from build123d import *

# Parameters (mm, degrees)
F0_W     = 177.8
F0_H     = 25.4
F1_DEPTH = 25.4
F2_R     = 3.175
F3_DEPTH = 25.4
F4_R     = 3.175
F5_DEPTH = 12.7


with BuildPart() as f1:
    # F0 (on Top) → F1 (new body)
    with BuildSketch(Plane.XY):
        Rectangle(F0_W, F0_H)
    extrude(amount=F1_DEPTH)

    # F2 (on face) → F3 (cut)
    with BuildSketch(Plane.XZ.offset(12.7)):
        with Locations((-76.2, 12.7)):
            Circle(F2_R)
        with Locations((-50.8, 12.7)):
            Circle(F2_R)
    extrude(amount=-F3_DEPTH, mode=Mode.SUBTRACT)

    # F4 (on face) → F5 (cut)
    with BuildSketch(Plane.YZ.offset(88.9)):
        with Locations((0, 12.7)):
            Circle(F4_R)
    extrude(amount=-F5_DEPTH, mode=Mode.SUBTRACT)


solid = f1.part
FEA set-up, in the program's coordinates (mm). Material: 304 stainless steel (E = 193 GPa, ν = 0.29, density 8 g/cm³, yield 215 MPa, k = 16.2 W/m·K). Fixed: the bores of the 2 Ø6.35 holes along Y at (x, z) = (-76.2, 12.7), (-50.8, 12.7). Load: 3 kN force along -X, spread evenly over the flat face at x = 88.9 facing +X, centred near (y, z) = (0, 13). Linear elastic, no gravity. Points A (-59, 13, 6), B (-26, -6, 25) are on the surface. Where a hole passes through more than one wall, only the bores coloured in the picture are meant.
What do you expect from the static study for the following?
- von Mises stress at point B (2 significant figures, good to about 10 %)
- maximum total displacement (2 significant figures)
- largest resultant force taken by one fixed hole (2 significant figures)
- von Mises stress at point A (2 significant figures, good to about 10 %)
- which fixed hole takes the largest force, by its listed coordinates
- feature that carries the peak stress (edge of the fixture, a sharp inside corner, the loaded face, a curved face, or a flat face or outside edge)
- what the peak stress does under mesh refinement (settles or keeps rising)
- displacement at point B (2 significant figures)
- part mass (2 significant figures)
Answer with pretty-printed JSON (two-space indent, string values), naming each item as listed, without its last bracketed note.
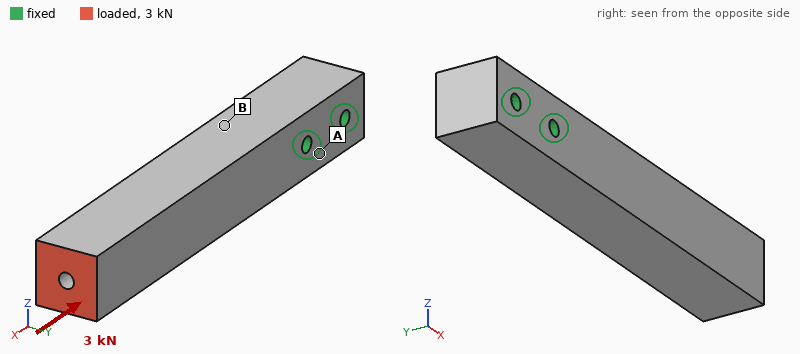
{
  "von Mises stress at point B": "4.6 MPa",
  "maximum total displacement": "3.5 µm",
  "largest resultant force taken by one fixed hole": "2.6 kN",
  "von Mises stress at point A": "1.6 MPa",
  "which fixed hole takes the largest force, by its listed coordinates": "(-50.8, 12.7)",
  "feature that carries the peak stress": "edge of the fixture",
  "what the peak stress does under mesh refinement": "keeps rising",
  "displacement at point B": "0.66 µm",
  "part mass": "900 g"
}
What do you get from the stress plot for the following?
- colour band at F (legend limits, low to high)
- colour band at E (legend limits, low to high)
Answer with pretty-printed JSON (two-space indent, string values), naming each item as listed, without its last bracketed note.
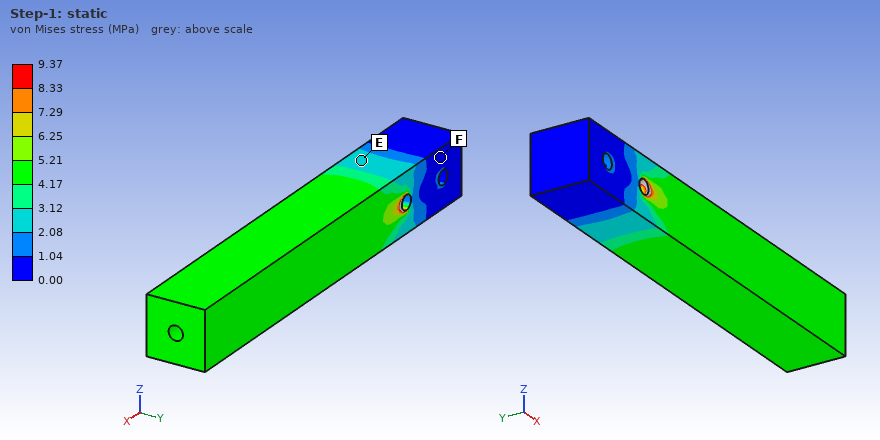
{
  "colour band at F": "0.00 to 1.04 MPa",
  "colour band at E": "2.08 to 3.12 MPa"
}
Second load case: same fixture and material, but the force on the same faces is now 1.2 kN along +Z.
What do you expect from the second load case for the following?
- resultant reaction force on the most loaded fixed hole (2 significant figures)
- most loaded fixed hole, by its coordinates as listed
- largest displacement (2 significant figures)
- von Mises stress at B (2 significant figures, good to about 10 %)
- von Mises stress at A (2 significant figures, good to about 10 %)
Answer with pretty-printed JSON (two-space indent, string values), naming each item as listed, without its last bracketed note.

{
  "resultant reaction force on the most loaded fixed hole": "5.2 kN",
  "most loaded fixed hole, by its coordinates as listed": "(-50.8, 12.7)",
  "largest displacement": "0.20 mm",
  "von Mises stress at B": "51 MPa",
  "von Mises stress at A": "20 MPa"
}
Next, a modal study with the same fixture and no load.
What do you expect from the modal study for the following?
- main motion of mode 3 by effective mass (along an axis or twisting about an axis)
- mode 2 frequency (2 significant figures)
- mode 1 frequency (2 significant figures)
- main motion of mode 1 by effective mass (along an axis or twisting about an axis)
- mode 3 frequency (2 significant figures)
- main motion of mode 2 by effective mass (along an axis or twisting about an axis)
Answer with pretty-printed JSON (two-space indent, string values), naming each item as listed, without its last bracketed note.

{
  "main motion of mode 3 by effective mass": "twisting about X",
  "mode 2 frequency": "1000 Hz",
  "mode 1 frequency": "910 Hz",
  "main motion of mode 1 by effective mass": "along Z",
  "mode 3 frequency": "5000 Hz",
  "main motion of mode 2 by effective mass": "along Y"
}
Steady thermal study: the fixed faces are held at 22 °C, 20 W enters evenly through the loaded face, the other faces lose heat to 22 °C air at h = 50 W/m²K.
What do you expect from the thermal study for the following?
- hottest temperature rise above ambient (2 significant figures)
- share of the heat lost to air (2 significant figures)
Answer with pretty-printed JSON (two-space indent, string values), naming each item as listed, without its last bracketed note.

{
  "hottest temperature rise above ambient": "85 K",
  "share of the heat lost to air": "91 %"
}
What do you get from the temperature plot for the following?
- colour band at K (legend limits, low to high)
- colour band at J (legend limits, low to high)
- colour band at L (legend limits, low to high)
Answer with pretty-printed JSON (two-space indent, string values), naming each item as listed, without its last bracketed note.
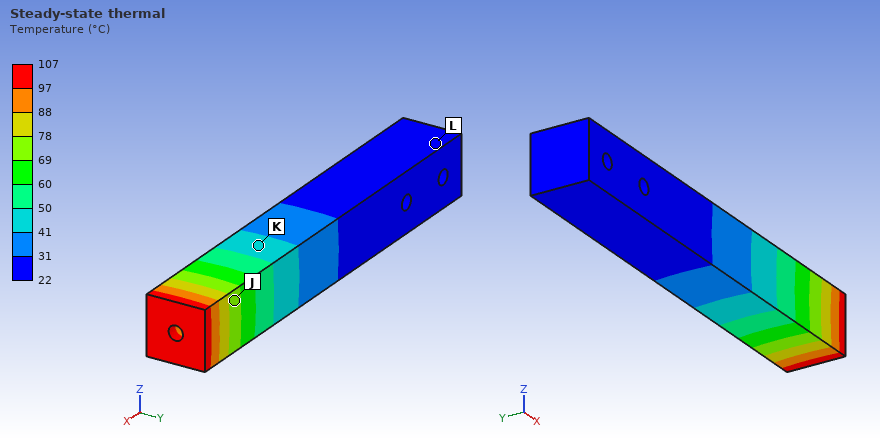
{
  "colour band at K": "41 to 50 °C",
  "colour band at J": "69 to 78 °C",
  "colour band at L": "22 to 31 °C"
}
